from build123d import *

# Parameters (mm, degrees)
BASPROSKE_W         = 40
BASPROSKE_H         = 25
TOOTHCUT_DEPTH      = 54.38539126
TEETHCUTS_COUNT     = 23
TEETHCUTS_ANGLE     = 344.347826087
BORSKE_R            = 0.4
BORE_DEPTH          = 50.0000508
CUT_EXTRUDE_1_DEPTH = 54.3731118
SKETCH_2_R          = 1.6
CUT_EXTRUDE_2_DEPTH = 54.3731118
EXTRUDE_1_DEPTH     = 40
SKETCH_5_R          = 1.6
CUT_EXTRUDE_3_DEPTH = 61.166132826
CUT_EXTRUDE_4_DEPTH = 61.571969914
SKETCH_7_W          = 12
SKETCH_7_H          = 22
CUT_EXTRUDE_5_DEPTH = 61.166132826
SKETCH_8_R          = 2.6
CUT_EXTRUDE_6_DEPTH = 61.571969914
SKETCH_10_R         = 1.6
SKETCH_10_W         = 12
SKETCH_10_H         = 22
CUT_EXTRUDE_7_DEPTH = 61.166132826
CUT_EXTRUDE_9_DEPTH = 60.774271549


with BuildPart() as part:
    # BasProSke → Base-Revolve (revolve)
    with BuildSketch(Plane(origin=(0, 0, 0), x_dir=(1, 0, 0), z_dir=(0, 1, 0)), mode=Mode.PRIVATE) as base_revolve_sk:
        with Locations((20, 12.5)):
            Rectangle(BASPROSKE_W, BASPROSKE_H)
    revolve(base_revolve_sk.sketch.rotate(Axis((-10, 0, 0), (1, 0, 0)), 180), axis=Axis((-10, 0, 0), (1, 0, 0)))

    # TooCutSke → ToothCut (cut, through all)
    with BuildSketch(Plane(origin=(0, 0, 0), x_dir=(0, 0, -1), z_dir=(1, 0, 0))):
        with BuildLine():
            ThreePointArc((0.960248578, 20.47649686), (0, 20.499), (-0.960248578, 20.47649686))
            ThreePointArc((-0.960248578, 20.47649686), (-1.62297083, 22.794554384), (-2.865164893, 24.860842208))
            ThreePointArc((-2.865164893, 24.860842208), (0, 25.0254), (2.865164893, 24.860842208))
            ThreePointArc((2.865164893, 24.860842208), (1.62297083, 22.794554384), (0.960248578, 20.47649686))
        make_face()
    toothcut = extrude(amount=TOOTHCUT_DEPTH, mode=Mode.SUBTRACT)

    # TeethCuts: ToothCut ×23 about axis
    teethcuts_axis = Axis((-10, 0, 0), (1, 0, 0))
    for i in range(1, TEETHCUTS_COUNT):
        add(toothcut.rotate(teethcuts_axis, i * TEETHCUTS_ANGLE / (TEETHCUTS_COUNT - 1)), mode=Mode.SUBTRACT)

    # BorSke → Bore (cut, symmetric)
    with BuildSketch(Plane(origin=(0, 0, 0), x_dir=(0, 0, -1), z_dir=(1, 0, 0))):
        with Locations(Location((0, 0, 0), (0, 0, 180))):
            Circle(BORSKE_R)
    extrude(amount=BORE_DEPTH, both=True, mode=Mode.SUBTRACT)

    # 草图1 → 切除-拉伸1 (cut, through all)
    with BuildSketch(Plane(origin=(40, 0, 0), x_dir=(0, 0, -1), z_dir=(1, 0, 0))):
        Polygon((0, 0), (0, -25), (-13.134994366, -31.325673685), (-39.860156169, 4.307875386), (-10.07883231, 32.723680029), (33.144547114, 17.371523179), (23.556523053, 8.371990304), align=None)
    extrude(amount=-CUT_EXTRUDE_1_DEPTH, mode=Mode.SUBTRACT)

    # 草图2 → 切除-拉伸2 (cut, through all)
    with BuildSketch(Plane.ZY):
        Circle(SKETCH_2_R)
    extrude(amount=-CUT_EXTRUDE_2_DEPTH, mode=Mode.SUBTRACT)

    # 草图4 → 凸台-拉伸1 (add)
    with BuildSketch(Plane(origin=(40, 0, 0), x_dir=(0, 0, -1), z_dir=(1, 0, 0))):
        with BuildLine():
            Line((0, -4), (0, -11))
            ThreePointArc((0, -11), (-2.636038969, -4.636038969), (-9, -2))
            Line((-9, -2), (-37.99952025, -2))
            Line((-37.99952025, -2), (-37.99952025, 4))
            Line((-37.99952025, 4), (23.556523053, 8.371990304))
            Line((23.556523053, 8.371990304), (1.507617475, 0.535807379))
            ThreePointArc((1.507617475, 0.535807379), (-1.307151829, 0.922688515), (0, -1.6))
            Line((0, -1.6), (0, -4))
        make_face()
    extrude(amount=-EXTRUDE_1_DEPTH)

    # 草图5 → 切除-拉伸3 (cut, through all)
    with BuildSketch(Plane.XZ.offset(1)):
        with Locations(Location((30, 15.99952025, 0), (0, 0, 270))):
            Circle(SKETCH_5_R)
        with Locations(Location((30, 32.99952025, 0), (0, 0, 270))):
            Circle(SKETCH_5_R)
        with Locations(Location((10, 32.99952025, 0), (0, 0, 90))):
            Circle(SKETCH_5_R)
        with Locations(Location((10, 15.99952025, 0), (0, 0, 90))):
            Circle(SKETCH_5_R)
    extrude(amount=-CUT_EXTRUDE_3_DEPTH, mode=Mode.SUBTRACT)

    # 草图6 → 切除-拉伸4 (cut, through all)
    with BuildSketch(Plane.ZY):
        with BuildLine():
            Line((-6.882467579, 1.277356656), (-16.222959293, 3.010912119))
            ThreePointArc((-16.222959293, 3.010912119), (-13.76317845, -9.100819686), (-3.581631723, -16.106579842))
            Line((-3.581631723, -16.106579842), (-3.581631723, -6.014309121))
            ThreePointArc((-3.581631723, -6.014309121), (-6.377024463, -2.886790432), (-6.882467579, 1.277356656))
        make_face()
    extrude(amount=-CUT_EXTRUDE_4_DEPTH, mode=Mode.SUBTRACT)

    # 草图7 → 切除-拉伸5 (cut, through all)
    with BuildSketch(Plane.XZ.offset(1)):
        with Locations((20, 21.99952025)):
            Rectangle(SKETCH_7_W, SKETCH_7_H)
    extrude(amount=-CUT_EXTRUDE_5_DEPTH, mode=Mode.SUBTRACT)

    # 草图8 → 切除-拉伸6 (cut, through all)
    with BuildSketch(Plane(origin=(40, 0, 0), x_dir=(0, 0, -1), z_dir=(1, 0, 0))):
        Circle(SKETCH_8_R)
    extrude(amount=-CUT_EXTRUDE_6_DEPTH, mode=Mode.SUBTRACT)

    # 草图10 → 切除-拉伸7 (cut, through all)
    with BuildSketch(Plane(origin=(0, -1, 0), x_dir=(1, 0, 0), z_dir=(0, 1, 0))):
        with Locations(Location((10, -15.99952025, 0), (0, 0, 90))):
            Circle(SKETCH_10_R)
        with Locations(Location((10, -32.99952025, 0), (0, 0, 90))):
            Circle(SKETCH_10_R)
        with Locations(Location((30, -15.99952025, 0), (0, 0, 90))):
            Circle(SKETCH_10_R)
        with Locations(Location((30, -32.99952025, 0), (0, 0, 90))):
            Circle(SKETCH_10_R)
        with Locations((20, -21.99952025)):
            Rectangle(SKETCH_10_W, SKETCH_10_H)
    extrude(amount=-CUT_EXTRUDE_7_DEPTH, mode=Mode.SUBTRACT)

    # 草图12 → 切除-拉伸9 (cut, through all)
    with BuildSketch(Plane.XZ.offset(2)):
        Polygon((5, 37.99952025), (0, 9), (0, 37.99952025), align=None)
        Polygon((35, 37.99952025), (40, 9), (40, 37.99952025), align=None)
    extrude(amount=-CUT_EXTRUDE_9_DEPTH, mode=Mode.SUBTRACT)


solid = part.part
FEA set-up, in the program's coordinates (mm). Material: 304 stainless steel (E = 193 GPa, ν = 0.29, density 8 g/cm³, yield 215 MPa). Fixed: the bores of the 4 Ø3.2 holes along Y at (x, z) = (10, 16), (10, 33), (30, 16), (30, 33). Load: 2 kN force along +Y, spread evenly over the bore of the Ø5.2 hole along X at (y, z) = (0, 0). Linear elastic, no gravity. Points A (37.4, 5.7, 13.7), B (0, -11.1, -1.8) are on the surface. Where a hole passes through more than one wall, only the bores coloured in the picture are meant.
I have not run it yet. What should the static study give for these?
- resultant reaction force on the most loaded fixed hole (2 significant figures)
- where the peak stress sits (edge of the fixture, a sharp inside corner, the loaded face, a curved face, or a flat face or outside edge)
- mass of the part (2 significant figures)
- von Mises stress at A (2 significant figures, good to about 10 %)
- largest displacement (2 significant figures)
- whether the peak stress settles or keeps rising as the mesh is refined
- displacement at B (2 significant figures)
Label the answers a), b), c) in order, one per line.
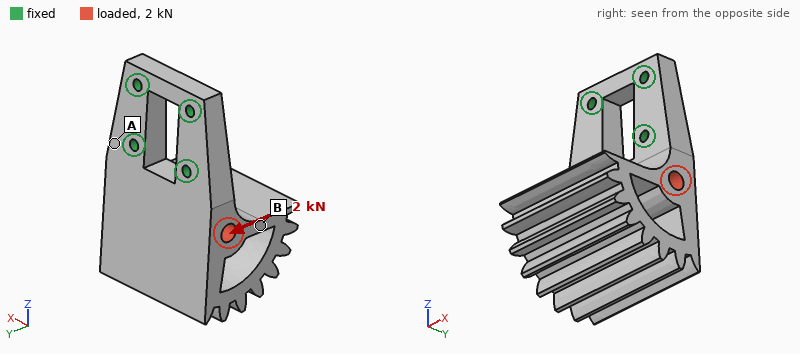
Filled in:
a) 1.2 kN
b) edge of the fixture
c) 190 g
d) 58 MPa
e) 49 µm
f) keeps rising
g) 25 µm
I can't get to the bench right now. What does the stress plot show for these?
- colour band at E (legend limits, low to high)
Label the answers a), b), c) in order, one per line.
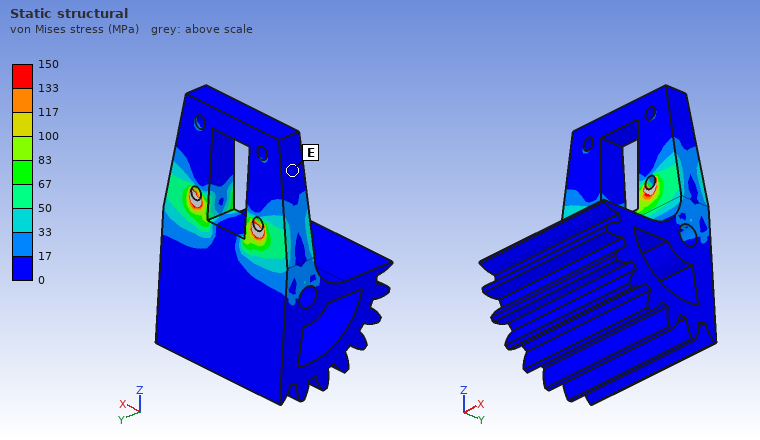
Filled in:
a) 0 to 17 MPa
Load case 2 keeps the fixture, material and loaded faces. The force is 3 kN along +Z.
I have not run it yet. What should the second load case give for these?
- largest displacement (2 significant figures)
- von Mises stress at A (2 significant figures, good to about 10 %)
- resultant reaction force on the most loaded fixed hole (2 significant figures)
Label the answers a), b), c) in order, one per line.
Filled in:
a) 13 µm
b) 8.0 MPa
c) 1.4 kN
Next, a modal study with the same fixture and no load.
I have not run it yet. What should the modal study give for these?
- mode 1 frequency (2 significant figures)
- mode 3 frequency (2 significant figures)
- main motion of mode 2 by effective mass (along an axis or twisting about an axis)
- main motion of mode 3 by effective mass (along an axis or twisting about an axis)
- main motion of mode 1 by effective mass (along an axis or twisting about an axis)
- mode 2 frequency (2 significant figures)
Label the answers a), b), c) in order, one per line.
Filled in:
a) 2100 Hz
b) 8100 Hz
c) along X
d) along X
e) along Y
f) 5400 Hz
